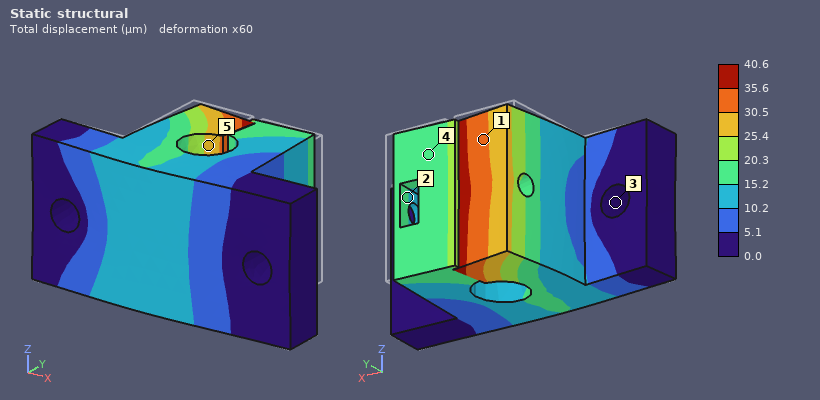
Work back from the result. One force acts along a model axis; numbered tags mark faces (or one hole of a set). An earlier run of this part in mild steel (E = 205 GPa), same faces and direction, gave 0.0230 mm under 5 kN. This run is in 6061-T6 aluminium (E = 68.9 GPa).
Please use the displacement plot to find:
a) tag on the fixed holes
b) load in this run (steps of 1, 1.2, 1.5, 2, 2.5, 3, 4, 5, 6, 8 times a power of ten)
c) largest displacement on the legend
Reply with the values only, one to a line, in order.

3
3 kN
40.6 µm
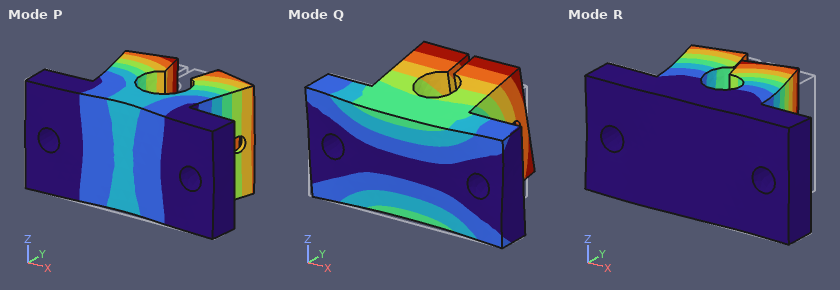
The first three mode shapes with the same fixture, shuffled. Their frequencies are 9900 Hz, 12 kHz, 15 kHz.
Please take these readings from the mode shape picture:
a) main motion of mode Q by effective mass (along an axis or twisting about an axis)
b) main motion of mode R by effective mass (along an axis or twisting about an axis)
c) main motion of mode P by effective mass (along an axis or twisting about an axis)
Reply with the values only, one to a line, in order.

along Z
along X
along Y
